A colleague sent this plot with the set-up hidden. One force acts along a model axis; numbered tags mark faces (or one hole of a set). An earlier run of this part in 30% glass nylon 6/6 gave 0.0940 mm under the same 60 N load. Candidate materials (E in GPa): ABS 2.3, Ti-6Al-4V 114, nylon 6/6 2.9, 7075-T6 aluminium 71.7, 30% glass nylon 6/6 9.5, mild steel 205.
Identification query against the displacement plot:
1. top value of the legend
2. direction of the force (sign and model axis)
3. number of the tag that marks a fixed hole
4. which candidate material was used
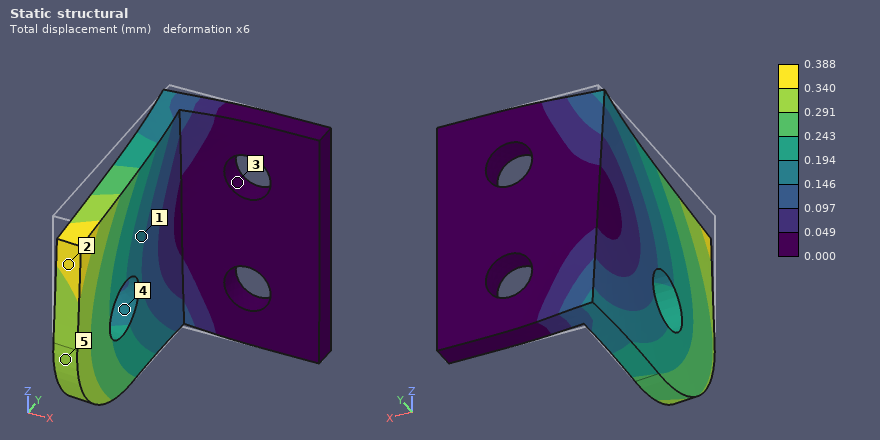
0.388 mm
-Z
3
ABS
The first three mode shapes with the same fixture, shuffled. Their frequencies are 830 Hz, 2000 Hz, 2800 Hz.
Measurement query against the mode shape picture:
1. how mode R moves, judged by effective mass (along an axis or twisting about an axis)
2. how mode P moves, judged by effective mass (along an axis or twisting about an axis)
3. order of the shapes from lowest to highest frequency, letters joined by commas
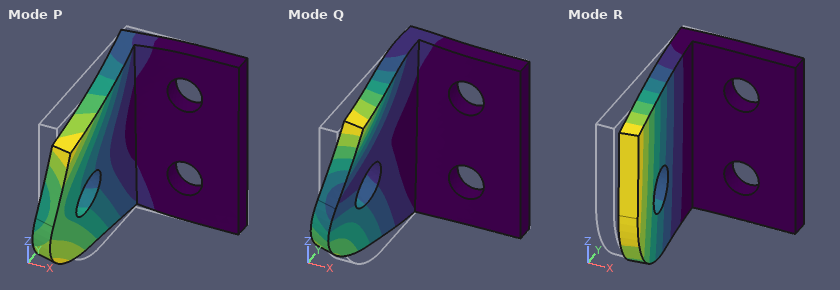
along X
along Z
R, P, Q
